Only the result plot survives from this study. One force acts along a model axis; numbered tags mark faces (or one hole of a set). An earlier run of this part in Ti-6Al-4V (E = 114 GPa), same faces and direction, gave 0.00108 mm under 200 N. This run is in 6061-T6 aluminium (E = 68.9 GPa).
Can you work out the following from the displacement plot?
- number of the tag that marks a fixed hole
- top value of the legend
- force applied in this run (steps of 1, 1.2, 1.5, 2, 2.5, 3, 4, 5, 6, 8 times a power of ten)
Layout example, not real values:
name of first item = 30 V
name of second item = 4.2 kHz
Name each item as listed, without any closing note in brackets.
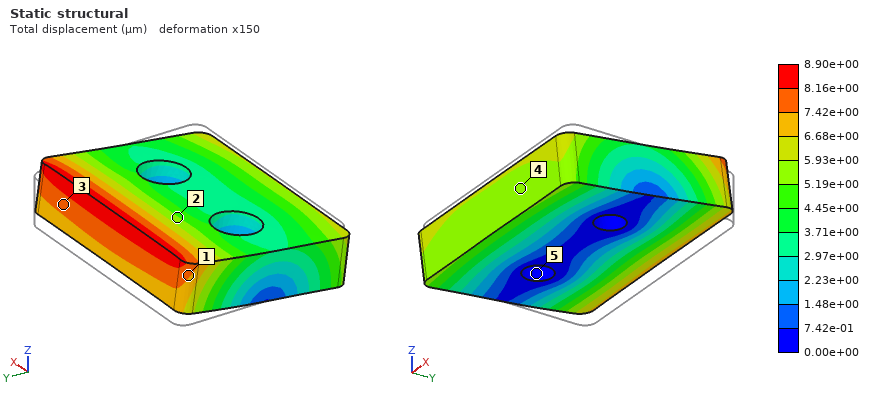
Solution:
number of the tag that marks a fixed hole = 5
top value of the legend = 8.90e+00 µm
force applied in this run = 1 kN
